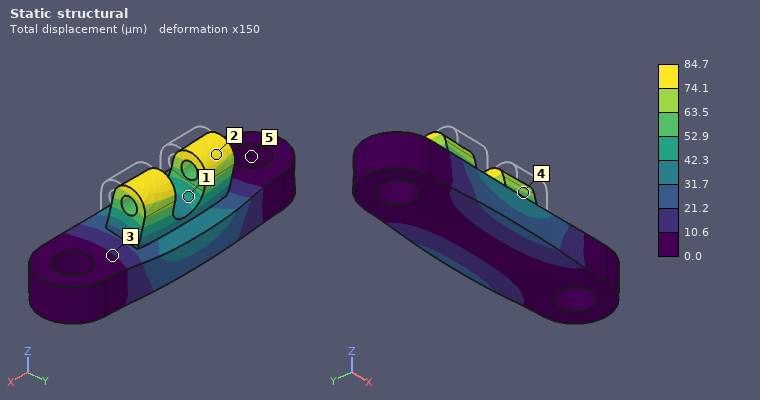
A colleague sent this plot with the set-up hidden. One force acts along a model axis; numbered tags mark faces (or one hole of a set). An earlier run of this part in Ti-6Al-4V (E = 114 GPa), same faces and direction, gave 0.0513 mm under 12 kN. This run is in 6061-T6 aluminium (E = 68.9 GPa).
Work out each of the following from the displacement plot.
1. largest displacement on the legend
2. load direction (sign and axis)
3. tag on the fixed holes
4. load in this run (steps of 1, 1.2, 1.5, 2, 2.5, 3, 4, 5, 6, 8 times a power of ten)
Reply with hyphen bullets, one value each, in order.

- 84.7 µm
- +Y
- 5
- 12 kN
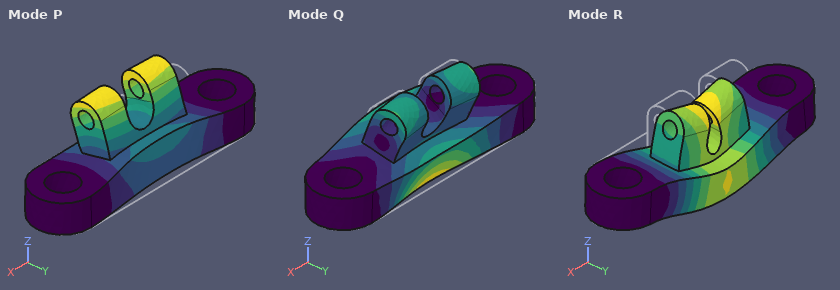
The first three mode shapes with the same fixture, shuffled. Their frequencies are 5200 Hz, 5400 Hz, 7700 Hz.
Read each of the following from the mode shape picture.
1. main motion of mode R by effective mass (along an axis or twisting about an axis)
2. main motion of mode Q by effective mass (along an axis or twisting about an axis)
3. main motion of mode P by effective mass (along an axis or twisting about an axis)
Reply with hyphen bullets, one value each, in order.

- along Z
- along Y
- along Y
